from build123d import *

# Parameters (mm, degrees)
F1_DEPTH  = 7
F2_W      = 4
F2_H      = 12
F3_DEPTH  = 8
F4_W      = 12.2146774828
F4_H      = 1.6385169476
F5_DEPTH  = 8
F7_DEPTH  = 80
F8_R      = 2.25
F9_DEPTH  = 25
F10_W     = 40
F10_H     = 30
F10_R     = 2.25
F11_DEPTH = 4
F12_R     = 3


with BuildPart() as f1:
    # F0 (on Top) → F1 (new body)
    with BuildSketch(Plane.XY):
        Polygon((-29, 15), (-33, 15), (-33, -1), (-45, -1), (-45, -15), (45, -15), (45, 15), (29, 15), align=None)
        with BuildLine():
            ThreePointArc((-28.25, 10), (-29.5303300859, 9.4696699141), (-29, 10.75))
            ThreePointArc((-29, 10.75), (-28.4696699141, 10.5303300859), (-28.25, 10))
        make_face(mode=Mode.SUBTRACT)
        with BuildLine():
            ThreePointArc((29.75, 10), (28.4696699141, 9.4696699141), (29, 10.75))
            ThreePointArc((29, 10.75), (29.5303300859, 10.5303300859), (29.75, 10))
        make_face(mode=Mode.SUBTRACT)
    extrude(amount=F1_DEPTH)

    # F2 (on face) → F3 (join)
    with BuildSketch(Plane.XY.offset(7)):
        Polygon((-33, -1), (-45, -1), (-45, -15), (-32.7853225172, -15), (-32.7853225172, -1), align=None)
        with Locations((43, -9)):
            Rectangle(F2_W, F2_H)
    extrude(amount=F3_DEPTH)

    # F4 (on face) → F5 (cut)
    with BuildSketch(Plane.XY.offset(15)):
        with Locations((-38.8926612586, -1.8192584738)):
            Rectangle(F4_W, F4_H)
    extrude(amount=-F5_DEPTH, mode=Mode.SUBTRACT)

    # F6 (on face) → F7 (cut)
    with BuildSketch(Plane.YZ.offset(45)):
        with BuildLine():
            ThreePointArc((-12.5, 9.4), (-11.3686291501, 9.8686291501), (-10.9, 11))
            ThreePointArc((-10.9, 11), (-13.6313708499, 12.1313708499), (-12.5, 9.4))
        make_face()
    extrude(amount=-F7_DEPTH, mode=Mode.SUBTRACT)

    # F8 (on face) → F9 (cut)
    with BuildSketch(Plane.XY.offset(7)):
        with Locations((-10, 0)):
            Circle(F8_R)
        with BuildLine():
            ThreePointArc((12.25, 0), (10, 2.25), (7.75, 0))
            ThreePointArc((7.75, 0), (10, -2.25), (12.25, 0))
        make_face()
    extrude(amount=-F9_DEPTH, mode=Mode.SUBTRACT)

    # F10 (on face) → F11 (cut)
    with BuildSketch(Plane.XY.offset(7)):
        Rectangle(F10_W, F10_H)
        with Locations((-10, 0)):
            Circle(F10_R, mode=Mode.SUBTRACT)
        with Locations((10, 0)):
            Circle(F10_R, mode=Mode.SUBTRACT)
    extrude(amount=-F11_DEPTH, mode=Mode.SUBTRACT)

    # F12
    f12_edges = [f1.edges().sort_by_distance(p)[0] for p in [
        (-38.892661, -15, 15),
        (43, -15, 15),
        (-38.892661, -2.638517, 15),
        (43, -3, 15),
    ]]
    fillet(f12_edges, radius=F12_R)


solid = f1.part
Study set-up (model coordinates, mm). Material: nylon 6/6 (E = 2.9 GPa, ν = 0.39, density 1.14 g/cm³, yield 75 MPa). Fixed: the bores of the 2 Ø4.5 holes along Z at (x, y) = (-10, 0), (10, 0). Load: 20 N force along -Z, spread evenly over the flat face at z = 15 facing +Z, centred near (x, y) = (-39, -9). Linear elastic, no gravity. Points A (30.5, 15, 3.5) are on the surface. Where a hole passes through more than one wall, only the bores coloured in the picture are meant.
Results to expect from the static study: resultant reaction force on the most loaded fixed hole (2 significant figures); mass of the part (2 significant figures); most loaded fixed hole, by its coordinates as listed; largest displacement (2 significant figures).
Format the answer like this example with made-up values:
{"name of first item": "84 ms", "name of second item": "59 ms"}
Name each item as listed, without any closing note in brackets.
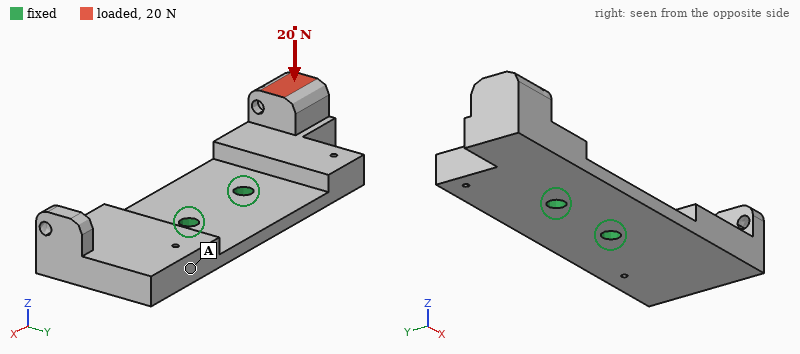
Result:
{"resultant reaction force on the most loaded fixed hole": "28 N", "mass of the part": "16 g", "most loaded fixed hole, by its coordinates as listed": "(-10, 0)", "largest displacement": "0.95 mm"}
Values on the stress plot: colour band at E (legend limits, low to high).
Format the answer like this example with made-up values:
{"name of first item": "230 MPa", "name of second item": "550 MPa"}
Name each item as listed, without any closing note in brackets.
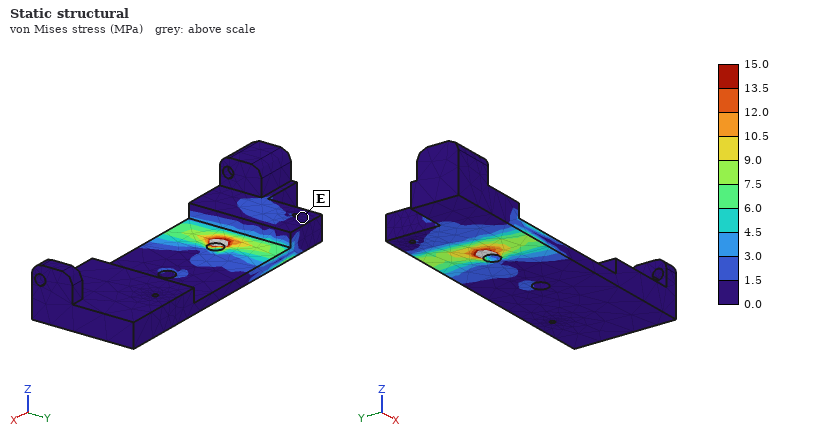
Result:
{"colour band at E": "0.0 to 1.5 MPa"}
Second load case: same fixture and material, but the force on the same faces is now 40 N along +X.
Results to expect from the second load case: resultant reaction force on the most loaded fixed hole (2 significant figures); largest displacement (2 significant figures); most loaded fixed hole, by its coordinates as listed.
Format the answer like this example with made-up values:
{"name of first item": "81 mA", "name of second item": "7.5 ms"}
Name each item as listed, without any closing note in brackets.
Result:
{"resultant reaction force on the most loaded fixed hole": "35 N", "largest displacement": "1.1 mm", "most loaded fixed hole, by its coordinates as listed": "(-10, 0)"}
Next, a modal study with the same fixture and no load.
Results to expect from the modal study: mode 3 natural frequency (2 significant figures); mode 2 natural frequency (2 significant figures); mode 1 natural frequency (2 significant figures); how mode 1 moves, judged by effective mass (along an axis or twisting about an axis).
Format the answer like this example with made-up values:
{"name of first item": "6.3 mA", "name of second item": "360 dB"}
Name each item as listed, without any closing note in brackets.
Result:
{"mode 3 natural frequency": "1200 Hz", "mode 2 natural frequency": "450 Hz", "mode 1 natural frequency": "430 Hz", "how mode 1 moves, judged by effective mass": "along Z"}
